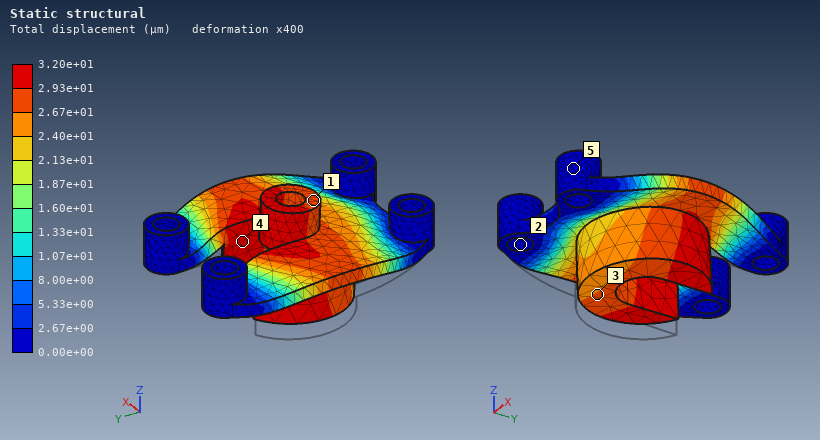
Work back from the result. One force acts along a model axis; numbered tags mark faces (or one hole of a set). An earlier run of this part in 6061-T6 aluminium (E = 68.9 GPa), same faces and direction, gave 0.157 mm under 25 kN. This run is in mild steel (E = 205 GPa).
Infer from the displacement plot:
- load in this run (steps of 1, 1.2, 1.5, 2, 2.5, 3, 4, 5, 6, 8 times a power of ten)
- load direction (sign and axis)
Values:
15 kN
+Z
